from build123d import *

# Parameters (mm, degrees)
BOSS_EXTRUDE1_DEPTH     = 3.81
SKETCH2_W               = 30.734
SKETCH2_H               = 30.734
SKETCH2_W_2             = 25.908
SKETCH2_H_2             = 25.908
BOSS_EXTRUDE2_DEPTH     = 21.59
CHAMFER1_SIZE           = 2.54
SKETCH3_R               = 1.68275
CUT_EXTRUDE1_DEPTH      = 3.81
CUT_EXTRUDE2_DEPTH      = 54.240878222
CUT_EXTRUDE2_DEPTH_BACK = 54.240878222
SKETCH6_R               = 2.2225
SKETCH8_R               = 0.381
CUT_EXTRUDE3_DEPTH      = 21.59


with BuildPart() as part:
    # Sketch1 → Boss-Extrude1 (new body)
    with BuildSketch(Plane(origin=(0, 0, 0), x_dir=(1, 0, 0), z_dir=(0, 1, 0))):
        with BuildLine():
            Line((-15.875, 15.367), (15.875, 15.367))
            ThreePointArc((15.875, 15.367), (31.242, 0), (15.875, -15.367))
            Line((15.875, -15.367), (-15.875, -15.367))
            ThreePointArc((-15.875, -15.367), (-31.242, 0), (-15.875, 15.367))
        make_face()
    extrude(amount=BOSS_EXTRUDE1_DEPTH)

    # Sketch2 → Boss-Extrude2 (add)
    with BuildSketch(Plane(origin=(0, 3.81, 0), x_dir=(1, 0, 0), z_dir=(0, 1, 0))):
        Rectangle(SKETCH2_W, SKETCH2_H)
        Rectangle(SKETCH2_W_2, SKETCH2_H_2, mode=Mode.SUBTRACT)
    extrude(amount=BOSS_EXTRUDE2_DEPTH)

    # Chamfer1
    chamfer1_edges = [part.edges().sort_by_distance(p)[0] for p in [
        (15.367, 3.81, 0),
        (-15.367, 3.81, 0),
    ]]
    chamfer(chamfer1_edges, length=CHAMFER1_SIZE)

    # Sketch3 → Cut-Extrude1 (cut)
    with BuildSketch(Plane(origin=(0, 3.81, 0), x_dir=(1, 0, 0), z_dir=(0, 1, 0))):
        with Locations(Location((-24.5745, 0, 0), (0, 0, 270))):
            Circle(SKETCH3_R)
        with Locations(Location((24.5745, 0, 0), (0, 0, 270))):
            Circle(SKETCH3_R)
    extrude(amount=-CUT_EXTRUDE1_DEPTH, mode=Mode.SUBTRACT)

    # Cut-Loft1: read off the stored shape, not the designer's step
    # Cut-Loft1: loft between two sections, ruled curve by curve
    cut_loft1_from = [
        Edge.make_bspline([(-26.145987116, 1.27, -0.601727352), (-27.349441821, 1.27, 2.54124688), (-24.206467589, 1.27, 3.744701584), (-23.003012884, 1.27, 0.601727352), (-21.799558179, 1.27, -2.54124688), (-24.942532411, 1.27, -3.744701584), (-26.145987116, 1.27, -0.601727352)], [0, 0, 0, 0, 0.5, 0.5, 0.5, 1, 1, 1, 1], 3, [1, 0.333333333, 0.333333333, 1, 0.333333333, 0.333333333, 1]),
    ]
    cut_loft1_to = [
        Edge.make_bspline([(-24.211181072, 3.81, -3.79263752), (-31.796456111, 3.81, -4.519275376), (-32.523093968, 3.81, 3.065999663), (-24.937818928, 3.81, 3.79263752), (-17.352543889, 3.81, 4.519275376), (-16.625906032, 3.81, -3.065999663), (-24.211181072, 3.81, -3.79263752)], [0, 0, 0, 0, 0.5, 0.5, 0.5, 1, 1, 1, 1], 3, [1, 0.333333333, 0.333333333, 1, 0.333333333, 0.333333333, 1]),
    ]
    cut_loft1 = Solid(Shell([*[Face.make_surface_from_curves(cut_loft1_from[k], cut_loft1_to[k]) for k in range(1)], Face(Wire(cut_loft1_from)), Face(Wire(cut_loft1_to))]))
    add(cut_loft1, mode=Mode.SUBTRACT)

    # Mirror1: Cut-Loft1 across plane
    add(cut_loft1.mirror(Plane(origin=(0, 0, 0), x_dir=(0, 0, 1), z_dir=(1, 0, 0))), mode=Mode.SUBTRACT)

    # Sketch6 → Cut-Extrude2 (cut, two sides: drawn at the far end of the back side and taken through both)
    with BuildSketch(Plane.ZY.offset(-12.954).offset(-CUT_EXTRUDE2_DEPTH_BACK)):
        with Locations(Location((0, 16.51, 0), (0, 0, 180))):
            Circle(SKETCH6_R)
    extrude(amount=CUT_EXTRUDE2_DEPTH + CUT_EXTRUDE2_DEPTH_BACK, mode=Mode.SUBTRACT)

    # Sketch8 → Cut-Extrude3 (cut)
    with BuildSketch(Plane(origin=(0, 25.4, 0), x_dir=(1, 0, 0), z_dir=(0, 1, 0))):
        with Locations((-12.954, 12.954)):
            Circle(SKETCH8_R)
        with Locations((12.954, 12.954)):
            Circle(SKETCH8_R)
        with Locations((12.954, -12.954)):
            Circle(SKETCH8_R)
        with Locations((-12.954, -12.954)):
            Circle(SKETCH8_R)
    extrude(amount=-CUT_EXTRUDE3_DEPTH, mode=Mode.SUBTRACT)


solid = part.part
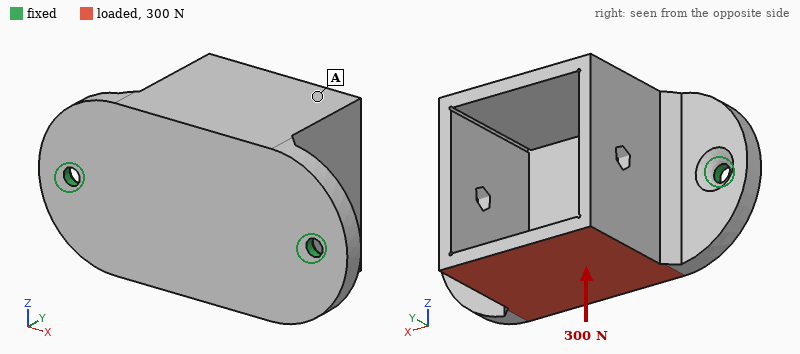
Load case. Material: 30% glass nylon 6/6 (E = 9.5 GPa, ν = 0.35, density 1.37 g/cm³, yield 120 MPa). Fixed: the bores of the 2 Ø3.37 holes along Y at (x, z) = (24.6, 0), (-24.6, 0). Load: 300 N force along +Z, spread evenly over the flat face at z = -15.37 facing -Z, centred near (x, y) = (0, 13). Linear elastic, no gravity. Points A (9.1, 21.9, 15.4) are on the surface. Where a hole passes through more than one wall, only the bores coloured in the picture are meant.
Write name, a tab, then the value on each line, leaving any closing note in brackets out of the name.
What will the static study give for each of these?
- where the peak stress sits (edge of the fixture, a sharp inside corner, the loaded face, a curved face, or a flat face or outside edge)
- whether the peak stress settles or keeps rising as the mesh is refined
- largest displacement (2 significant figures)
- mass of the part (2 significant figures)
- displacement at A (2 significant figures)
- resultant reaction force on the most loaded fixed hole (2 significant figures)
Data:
where the peak stress sits	edge of the fixture
whether the peak stress settles or keeps rising as the mesh is refined	keeps rising
largest displacement	0.67 mm
mass of the part	17 g
displacement at A	0.49 mm
resultant reaction force on the most loaded fixed hole	150 N
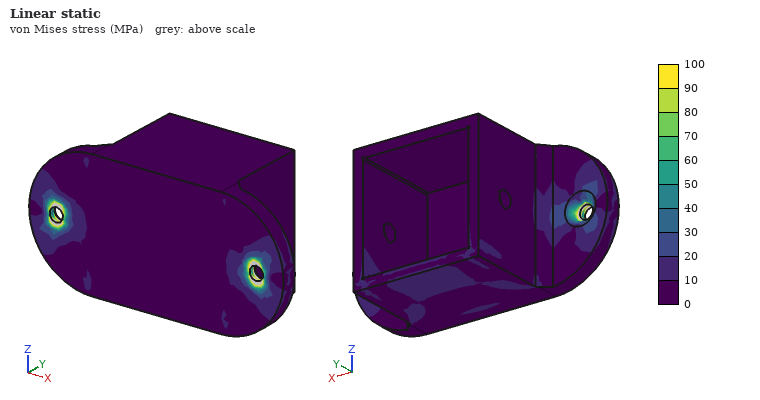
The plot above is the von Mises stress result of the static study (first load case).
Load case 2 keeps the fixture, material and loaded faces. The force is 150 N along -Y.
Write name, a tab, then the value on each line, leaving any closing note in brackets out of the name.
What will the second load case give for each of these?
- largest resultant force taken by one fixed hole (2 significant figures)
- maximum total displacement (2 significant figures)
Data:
largest resultant force taken by one fixed hole	100 N
maximum total displacement	0.39 mm
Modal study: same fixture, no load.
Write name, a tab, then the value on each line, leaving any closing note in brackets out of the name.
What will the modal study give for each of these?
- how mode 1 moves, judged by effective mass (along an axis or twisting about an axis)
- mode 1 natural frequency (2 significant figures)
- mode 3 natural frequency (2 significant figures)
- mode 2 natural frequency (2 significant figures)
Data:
how mode 1 moves, judged by effective mass	along Z
mode 1 natural frequency	1200 Hz
mode 3 natural frequency	3300 Hz
mode 2 natural frequency	3300 Hz
